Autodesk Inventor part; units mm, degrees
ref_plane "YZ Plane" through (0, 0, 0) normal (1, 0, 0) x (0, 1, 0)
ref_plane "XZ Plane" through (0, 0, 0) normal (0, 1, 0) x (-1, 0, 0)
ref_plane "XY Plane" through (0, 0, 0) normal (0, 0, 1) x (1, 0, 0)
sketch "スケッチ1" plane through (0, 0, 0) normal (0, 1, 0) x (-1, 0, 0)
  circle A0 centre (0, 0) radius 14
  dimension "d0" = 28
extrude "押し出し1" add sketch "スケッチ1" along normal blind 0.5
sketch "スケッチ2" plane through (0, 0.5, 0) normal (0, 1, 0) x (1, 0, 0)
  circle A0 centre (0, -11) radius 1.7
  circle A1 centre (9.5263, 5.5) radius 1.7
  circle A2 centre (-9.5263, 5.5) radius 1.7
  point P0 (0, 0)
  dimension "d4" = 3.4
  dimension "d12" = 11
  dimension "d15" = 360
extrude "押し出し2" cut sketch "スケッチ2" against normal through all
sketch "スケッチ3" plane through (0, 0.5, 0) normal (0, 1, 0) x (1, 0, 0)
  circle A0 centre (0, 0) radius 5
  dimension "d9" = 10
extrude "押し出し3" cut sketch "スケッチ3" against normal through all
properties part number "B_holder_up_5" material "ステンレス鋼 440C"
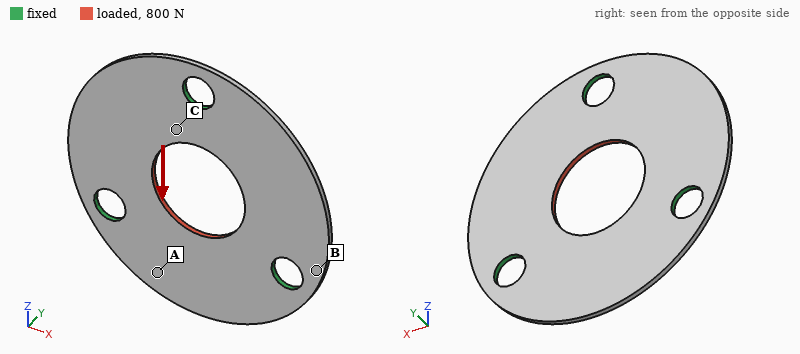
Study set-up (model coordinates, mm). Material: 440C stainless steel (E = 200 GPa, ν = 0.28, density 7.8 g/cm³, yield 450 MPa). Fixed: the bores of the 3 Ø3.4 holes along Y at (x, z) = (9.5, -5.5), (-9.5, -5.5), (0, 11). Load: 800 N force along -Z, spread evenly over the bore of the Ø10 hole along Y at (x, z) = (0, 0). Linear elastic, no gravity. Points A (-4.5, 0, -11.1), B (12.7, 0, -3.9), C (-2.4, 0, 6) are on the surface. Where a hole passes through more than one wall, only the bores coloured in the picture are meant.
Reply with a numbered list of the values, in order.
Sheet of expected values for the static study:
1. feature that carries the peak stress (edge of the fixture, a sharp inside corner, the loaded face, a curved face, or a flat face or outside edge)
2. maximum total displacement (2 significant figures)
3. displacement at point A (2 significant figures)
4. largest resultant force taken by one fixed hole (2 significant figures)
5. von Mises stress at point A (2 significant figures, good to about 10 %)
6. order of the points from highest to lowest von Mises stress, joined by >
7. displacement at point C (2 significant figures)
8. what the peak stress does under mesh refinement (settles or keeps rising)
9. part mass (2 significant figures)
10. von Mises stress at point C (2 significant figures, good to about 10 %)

1. edge of the fixture
2. 4.4 µm
3. 2.5 µm
4. 280 N
5. 40 MPa
6. C > A > B
7. 1.6 µm
8. keeps rising
9. 2.0 g
10. 72 MPa
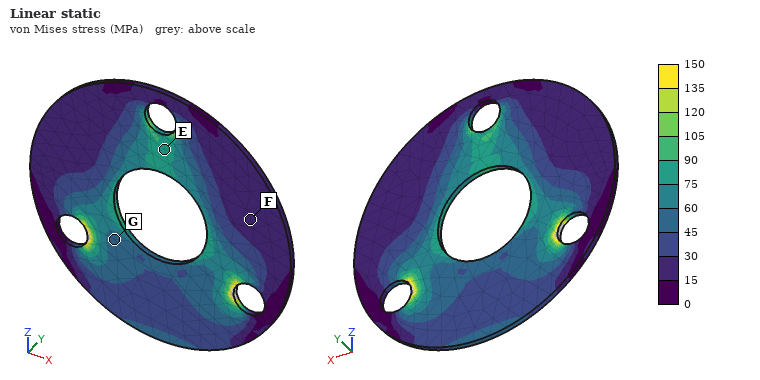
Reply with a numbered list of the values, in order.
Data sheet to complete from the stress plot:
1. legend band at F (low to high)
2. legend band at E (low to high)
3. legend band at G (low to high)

1. 15 to 30 MPa
2. 75 to 90 MPa
3. 45 to 60 MPa
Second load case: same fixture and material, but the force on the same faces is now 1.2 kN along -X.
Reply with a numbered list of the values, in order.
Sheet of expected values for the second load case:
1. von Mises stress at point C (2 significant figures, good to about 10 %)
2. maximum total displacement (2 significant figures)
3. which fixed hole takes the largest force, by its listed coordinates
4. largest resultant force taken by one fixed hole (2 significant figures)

1. 76 MPa
2. 5.9 µm
3. (0, 11)
4. 440 N
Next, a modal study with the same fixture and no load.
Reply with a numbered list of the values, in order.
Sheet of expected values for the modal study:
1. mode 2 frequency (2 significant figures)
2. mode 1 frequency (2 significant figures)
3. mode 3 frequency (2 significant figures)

1. 5800 Hz
2. 5800 Hz
3. 5900 Hz
